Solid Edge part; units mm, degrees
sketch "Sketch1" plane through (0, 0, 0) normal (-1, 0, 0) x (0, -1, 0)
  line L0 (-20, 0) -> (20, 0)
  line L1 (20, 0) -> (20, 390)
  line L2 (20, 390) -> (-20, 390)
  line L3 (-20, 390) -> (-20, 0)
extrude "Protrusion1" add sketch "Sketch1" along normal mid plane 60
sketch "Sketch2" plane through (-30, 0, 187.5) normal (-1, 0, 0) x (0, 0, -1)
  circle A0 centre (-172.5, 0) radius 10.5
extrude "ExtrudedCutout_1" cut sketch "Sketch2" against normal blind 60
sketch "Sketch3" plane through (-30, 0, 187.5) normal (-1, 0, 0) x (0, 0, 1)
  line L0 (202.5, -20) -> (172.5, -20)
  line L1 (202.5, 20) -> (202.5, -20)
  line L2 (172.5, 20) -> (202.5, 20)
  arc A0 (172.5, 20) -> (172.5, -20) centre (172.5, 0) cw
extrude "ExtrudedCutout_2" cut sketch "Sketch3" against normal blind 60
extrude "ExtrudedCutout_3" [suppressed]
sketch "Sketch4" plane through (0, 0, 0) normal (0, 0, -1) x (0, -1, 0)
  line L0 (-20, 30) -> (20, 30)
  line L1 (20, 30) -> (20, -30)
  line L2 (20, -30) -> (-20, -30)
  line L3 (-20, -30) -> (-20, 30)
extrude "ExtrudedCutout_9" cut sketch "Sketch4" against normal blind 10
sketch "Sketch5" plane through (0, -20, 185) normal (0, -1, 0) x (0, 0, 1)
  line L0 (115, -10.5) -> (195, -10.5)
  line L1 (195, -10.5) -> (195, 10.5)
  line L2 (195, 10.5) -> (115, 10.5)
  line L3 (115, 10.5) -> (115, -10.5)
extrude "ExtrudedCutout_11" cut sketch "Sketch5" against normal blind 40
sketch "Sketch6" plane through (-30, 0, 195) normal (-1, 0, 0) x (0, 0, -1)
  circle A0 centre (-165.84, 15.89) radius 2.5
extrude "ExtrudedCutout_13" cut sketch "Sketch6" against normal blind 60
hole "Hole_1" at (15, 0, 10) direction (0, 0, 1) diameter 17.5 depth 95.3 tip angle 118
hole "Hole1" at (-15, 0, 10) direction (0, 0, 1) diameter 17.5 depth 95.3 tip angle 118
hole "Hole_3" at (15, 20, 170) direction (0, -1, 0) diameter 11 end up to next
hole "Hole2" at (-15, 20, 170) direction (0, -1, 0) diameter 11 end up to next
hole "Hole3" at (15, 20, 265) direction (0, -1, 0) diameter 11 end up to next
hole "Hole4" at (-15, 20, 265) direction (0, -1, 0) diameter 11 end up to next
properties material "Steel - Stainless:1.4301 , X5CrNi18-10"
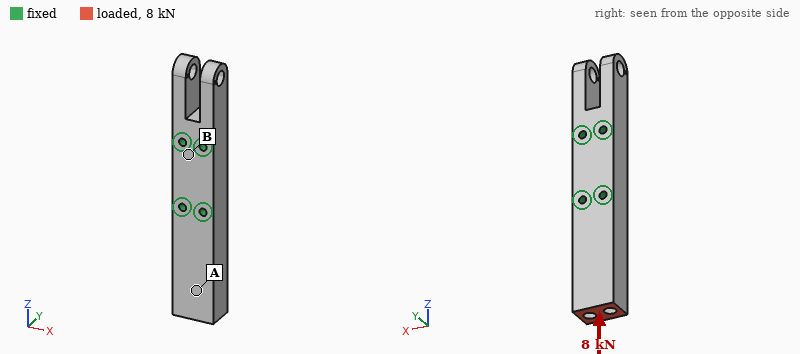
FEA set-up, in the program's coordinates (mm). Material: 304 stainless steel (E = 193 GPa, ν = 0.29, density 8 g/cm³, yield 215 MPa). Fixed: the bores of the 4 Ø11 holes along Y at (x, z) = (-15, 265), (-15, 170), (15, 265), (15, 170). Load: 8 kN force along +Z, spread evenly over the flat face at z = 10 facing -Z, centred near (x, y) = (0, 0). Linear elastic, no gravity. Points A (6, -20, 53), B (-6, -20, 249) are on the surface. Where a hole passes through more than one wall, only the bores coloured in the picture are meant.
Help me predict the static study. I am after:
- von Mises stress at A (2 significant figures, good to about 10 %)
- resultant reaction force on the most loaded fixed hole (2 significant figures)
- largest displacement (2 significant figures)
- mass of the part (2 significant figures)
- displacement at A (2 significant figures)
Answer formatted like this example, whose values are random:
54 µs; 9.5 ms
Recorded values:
4.2 MPa; 3.9 kN; 3.2 µm; 5.9 kg; 2.3 µm
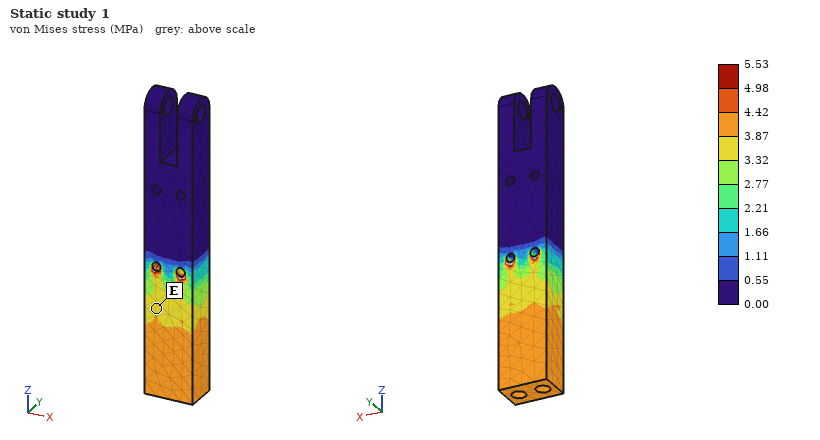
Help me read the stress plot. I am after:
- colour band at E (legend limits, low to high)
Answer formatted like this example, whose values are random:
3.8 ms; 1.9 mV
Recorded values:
3.32 to 3.87 MPa
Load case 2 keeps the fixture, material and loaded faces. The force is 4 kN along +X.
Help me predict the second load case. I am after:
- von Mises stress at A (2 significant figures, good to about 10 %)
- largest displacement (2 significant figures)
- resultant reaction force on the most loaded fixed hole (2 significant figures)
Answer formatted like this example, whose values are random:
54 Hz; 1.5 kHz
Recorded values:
6.1 MPa; 50 µm; 16 kN
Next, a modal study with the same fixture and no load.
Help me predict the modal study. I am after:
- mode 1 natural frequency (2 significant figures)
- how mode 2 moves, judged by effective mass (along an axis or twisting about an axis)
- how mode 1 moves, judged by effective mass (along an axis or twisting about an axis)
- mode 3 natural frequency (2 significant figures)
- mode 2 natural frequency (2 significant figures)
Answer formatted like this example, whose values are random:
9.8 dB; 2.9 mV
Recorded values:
1300 Hz; along X; along Y; 2200 Hz; 1800 Hz
